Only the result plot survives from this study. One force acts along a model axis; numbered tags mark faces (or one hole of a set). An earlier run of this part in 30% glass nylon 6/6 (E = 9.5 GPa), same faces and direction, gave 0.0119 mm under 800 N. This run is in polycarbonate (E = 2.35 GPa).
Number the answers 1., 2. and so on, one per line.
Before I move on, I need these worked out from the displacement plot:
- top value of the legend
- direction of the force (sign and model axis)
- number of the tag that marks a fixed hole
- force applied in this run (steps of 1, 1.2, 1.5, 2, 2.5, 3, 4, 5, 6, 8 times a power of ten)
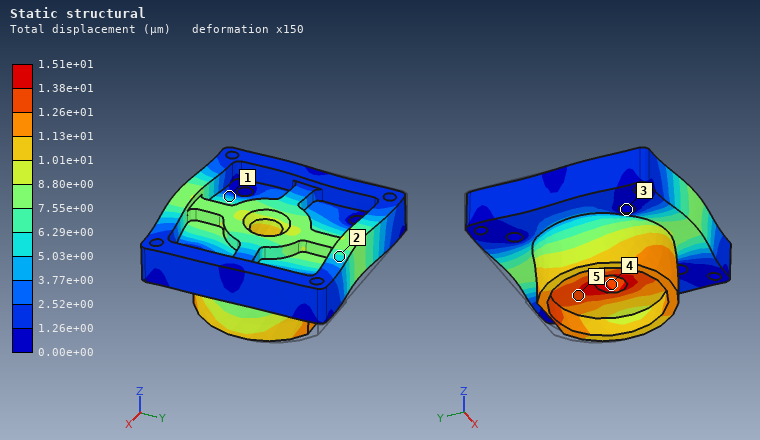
1. 1.51e+01 µm
2. -Y
3. 3
4. 250 N
